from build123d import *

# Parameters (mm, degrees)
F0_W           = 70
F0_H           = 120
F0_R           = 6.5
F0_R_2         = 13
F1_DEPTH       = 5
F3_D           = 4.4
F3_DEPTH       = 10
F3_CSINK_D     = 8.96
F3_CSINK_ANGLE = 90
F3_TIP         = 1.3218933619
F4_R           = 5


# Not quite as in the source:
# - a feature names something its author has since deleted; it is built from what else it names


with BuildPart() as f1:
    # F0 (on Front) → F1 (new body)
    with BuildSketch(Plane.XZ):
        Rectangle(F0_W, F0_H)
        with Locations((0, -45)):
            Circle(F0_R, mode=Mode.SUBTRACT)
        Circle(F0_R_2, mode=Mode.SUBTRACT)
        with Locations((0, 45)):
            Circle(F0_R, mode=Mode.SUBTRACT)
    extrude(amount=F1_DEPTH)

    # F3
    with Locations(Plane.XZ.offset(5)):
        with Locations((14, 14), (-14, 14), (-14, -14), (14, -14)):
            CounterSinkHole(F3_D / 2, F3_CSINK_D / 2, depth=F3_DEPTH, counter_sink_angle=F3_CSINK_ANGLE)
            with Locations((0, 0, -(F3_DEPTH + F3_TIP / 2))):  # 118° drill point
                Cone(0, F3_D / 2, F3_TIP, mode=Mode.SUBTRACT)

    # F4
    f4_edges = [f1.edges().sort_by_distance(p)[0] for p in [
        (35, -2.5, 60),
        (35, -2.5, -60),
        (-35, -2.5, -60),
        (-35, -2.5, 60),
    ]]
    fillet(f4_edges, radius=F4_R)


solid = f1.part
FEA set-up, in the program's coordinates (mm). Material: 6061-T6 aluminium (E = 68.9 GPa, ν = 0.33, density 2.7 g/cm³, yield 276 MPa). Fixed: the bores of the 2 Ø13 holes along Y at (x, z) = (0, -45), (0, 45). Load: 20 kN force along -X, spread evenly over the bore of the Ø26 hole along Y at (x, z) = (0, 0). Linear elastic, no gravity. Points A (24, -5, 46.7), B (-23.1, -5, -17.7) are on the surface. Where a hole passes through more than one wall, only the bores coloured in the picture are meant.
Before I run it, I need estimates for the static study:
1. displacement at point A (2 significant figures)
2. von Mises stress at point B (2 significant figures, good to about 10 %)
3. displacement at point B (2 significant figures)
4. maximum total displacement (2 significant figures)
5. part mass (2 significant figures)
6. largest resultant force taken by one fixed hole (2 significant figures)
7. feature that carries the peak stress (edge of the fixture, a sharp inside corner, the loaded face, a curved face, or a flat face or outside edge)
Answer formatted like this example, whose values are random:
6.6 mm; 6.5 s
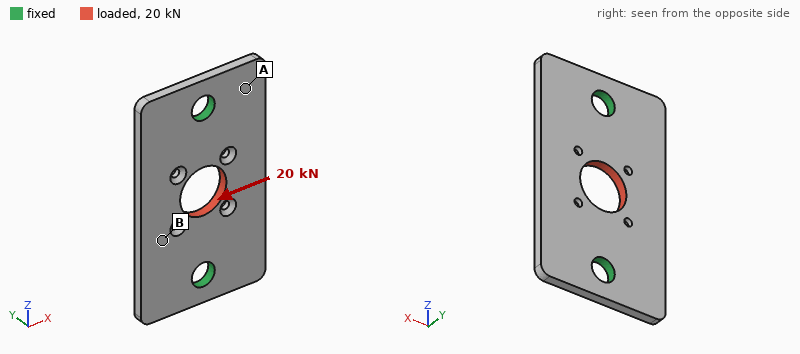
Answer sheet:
17 µm; 56 MPa; 52 µm; 77 µm; 100 g; 10 kN; edge of the fixture
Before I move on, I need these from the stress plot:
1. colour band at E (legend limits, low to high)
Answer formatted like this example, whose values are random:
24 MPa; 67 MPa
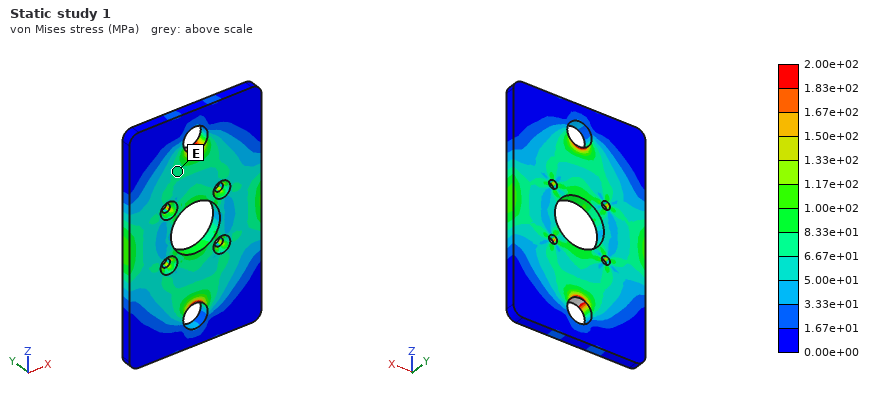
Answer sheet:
6.67e+01 to 8.33e+01 MPa
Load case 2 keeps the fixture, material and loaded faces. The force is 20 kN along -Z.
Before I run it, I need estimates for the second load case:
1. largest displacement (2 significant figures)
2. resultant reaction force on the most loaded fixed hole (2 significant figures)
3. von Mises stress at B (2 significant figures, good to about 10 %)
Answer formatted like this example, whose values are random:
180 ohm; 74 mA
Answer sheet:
38 µm; 10 kN; 26 MPa
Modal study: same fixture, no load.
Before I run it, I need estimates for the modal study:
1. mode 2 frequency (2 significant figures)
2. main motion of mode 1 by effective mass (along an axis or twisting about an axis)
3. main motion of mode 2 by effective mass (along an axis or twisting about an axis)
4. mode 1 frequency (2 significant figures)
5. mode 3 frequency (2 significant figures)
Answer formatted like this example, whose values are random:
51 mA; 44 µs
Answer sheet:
2800 Hz; twisting about Z; along Y; 2600 Hz; 4600 Hz
